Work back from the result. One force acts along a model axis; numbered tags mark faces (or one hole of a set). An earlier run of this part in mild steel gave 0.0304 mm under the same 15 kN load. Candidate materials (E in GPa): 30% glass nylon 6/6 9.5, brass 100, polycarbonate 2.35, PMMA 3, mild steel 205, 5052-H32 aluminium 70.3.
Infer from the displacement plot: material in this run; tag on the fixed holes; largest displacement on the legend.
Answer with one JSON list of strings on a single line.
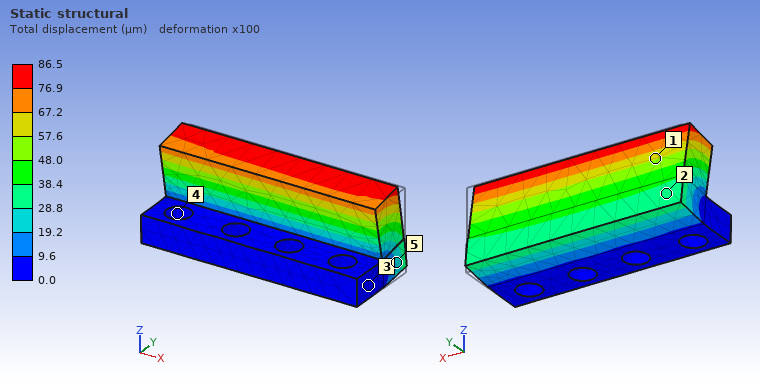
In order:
["5052-H32 aluminium", "4", "86.5 µm"]
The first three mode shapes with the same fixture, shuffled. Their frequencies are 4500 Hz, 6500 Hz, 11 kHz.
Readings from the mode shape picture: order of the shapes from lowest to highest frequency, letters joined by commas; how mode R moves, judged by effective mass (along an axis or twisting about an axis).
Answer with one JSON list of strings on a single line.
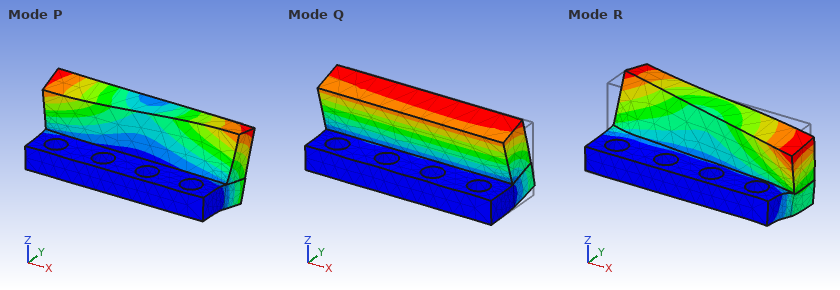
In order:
["Q, P, R", "along X"]
